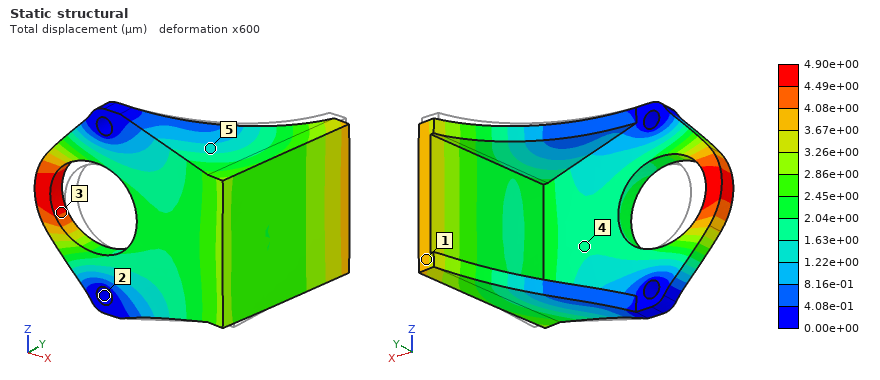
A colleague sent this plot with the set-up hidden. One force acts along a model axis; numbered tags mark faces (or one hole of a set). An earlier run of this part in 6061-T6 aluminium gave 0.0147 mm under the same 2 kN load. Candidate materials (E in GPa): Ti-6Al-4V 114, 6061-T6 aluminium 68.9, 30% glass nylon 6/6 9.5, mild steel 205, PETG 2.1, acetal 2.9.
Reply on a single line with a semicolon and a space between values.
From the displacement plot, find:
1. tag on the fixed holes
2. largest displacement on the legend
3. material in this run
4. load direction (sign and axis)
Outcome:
2; 4.90e+00 µm; mild steel; -X
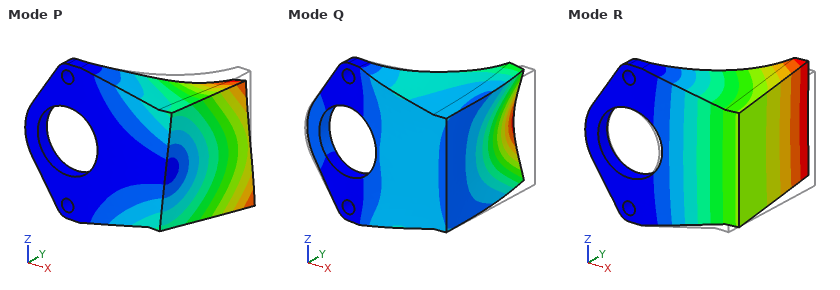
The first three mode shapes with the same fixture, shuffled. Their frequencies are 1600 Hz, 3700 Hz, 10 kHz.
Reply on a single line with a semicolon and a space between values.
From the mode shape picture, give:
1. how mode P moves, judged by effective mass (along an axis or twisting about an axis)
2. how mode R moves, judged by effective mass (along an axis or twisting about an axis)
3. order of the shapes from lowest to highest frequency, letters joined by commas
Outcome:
along Z; along Y; R, P, Q
